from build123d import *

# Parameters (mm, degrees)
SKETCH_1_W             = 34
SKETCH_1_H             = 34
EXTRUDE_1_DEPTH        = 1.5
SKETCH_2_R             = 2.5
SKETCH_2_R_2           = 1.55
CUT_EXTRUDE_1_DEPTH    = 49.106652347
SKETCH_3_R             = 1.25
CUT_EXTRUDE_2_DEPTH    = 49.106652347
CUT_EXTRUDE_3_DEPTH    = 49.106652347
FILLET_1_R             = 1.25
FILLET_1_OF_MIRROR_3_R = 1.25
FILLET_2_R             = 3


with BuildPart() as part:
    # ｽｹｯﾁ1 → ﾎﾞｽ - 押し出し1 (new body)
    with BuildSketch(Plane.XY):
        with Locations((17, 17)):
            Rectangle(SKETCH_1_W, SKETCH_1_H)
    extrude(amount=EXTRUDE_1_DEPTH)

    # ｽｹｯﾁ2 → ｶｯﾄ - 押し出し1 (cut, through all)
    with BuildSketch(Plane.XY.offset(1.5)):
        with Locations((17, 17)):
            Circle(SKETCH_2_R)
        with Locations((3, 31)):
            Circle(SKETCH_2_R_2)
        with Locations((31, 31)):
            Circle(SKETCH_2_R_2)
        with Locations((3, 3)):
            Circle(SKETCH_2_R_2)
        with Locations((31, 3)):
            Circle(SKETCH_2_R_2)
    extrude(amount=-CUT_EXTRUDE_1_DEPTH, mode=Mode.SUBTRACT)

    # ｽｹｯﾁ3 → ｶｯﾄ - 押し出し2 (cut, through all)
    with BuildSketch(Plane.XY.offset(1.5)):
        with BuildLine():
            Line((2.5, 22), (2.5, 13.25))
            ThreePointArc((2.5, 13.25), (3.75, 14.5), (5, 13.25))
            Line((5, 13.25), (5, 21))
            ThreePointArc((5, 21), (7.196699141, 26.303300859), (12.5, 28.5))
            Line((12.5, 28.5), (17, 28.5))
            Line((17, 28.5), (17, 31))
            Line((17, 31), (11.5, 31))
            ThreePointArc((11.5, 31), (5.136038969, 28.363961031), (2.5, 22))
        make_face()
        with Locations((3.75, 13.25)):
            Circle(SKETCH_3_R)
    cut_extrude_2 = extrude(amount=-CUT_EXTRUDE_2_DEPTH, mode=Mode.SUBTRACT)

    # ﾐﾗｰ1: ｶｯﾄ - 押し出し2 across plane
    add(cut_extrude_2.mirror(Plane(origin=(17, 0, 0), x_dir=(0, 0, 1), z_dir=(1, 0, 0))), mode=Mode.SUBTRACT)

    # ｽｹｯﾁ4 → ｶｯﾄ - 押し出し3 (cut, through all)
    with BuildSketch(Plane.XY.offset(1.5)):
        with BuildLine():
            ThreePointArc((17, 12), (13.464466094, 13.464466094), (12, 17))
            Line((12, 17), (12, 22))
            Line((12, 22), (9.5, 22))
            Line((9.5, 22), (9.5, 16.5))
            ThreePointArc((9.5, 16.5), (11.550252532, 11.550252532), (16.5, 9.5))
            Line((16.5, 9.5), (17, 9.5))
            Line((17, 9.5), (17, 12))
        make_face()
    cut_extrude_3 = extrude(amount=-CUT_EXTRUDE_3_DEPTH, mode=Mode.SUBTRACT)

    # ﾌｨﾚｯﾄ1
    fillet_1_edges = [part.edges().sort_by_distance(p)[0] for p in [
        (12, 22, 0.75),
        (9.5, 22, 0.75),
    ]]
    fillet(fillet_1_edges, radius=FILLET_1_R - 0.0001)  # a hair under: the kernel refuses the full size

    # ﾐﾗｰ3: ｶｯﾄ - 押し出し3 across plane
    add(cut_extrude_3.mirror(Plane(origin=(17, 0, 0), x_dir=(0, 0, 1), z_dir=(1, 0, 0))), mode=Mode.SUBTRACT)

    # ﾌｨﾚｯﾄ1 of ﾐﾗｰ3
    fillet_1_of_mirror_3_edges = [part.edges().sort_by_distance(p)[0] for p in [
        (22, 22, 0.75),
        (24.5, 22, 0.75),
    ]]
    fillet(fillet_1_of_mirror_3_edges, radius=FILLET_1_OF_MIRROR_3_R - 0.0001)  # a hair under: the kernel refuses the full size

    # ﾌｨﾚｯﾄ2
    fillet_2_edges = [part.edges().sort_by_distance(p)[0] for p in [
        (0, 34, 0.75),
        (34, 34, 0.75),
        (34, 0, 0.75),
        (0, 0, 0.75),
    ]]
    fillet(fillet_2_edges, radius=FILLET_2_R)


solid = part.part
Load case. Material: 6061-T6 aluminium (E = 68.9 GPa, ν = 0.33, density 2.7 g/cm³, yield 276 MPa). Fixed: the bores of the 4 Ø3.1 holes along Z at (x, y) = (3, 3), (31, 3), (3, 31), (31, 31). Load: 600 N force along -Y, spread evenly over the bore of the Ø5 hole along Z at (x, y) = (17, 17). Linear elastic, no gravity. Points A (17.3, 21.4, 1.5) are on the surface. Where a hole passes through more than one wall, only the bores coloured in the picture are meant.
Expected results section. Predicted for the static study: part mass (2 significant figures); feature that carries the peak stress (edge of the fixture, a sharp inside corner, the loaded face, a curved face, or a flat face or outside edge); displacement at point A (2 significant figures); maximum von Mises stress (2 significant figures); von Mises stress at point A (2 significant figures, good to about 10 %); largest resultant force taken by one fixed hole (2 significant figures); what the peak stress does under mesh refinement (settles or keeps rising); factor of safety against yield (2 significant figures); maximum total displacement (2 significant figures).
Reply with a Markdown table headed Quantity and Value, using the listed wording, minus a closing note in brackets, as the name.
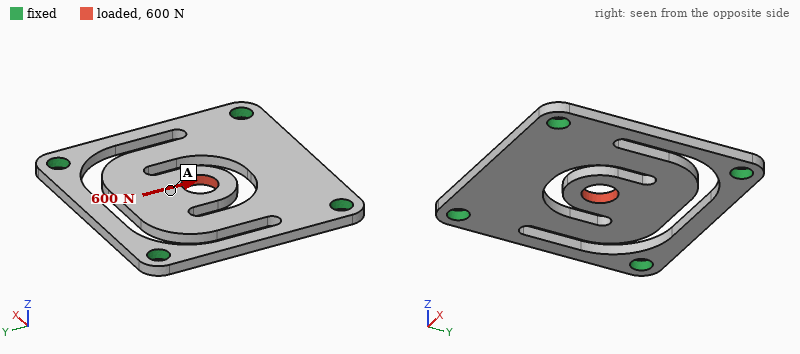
| Quantity | Value |
|---|---|
| part mass | 3.6 g |
| feature that carries the peak stress | a curved face |
| displacement at point A | 27 µm |
| maximum von Mises stress | 210 MPa |
| von Mises stress at point A | 22 MPa |
| largest resultant force taken by one fixed hole | 300 N |
| what the peak stress does under mesh refinement | settles |
| factor of safety against yield | 1.3 |
| maximum total displacement | 33 µm |
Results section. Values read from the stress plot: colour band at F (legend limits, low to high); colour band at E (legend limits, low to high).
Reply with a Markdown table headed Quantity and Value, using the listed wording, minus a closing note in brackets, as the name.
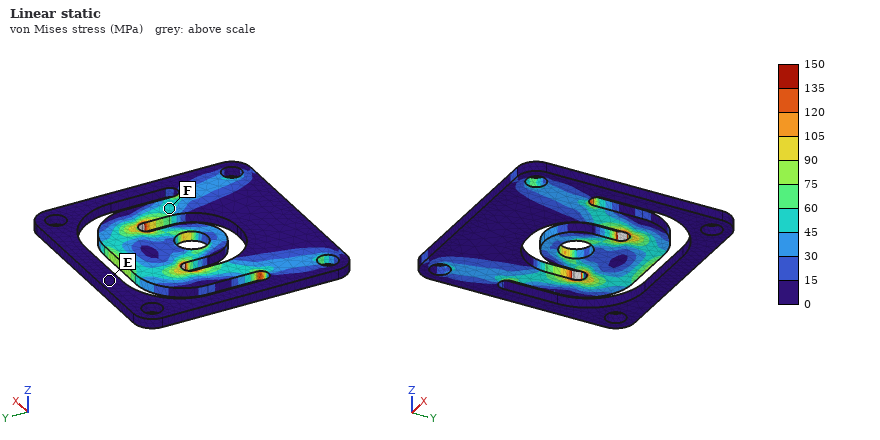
| Quantity | Value |
|---|---|
| colour band at F | 45 to 60 MPa |
| colour band at E | 0 to 15 MPa |
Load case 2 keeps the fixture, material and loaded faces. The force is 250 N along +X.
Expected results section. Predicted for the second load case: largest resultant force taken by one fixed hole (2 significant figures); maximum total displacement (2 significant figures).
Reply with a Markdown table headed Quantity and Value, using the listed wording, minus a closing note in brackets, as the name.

| Quantity | Value |
|---|---|
| largest resultant force taken by one fixed hole | 150 N |
| maximum total displacement | 75 µm |
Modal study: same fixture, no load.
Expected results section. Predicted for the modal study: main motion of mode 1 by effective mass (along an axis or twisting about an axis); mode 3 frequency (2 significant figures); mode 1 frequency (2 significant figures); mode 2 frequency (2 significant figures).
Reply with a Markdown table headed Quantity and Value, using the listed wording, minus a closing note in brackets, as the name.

| Quantity | Value |
|---|---|
| main motion of mode 1 by effective mass | along Z |
| mode 3 frequency | 5400 Hz |
| mode 1 frequency | 1900 Hz |
| mode 2 frequency | 5300 Hz |
